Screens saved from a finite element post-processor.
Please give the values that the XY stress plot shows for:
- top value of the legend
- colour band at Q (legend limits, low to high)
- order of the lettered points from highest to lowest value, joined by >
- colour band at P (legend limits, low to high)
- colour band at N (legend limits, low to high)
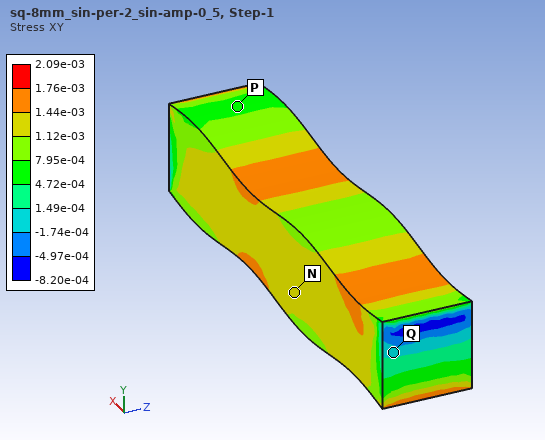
2.09e-03
-1.74e-04 to 1.49e-04
N > P > Q
4.72e-04 to 7.95e-04
1.12e-03 to 1.44e-03
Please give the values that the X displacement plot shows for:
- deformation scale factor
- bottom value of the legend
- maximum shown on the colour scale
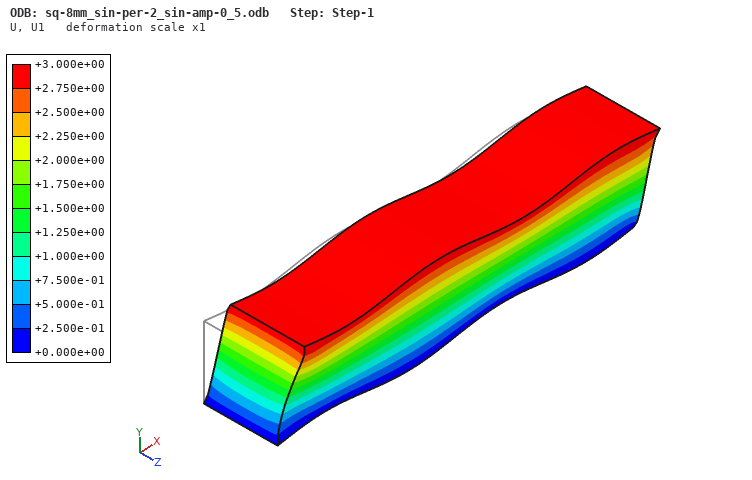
1
+0.000e+00
+3.000e+00
